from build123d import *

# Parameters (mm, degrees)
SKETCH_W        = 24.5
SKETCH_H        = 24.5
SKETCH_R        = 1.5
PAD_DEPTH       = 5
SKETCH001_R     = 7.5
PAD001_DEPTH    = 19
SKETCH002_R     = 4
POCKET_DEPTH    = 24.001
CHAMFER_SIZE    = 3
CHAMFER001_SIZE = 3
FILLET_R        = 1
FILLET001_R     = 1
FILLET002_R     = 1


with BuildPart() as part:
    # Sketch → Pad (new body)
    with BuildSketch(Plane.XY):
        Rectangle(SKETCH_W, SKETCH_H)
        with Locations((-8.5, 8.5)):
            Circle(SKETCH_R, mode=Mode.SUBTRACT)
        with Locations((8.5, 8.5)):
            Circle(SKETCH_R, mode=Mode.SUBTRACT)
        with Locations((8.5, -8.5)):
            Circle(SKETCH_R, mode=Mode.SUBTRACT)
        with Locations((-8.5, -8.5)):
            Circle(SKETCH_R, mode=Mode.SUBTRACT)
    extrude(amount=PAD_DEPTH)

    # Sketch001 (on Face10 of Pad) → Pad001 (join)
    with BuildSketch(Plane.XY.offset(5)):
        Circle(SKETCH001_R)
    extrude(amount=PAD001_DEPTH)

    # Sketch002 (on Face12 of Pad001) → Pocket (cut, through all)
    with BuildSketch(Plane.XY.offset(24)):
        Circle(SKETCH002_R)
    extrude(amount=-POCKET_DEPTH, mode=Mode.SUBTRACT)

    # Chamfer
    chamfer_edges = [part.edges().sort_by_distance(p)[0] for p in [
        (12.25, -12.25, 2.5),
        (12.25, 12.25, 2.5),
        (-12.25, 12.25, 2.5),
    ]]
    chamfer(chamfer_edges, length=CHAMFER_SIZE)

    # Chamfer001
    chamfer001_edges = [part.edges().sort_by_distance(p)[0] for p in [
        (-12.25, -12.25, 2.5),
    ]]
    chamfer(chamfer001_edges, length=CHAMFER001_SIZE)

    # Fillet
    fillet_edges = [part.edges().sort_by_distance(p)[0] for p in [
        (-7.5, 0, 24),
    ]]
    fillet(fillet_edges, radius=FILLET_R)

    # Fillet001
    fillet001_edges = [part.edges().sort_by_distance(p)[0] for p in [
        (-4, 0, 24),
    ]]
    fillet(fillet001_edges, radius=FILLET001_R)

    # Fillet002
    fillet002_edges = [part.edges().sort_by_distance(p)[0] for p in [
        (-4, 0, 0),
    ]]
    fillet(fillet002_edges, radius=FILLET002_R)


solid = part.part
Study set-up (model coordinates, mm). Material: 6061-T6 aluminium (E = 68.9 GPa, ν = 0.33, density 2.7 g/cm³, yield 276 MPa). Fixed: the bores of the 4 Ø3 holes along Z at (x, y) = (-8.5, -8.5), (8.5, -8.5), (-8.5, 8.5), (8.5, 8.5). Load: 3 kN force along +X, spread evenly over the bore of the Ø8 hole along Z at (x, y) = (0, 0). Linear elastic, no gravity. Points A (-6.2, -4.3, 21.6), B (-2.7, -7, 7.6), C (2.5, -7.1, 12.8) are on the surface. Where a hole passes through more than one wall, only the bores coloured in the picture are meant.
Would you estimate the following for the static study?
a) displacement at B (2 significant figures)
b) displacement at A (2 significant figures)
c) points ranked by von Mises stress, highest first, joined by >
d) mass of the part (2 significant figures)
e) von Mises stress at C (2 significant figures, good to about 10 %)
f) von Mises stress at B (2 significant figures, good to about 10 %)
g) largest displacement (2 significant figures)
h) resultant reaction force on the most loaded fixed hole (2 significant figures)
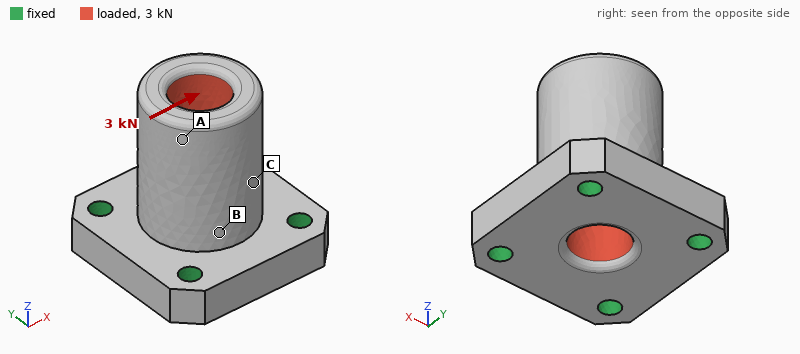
9.9 µm
44 µm
B > C > A
13 g
26 MPa
36 MPa
49 µm
1.2 kN
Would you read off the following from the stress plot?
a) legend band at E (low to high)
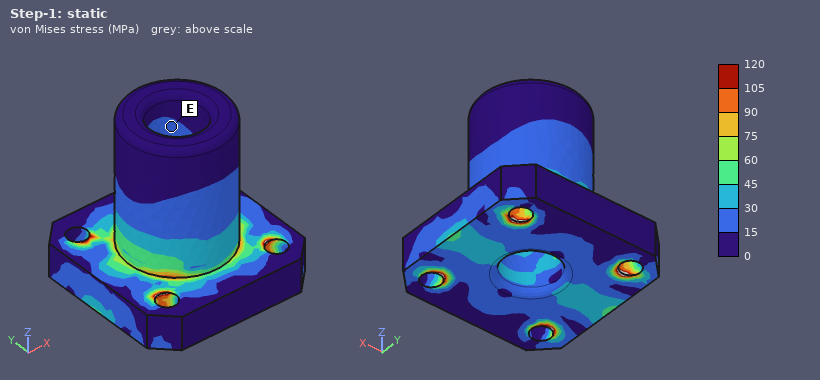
15 to 30 MPa
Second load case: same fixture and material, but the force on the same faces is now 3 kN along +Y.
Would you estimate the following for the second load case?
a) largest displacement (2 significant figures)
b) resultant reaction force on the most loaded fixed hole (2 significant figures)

49 µm
1.2 kN
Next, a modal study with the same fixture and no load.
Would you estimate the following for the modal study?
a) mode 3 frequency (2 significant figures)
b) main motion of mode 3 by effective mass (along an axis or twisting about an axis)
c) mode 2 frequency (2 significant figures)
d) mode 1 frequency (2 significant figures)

34 kHz
along Z
16 kHz
16 kHz
